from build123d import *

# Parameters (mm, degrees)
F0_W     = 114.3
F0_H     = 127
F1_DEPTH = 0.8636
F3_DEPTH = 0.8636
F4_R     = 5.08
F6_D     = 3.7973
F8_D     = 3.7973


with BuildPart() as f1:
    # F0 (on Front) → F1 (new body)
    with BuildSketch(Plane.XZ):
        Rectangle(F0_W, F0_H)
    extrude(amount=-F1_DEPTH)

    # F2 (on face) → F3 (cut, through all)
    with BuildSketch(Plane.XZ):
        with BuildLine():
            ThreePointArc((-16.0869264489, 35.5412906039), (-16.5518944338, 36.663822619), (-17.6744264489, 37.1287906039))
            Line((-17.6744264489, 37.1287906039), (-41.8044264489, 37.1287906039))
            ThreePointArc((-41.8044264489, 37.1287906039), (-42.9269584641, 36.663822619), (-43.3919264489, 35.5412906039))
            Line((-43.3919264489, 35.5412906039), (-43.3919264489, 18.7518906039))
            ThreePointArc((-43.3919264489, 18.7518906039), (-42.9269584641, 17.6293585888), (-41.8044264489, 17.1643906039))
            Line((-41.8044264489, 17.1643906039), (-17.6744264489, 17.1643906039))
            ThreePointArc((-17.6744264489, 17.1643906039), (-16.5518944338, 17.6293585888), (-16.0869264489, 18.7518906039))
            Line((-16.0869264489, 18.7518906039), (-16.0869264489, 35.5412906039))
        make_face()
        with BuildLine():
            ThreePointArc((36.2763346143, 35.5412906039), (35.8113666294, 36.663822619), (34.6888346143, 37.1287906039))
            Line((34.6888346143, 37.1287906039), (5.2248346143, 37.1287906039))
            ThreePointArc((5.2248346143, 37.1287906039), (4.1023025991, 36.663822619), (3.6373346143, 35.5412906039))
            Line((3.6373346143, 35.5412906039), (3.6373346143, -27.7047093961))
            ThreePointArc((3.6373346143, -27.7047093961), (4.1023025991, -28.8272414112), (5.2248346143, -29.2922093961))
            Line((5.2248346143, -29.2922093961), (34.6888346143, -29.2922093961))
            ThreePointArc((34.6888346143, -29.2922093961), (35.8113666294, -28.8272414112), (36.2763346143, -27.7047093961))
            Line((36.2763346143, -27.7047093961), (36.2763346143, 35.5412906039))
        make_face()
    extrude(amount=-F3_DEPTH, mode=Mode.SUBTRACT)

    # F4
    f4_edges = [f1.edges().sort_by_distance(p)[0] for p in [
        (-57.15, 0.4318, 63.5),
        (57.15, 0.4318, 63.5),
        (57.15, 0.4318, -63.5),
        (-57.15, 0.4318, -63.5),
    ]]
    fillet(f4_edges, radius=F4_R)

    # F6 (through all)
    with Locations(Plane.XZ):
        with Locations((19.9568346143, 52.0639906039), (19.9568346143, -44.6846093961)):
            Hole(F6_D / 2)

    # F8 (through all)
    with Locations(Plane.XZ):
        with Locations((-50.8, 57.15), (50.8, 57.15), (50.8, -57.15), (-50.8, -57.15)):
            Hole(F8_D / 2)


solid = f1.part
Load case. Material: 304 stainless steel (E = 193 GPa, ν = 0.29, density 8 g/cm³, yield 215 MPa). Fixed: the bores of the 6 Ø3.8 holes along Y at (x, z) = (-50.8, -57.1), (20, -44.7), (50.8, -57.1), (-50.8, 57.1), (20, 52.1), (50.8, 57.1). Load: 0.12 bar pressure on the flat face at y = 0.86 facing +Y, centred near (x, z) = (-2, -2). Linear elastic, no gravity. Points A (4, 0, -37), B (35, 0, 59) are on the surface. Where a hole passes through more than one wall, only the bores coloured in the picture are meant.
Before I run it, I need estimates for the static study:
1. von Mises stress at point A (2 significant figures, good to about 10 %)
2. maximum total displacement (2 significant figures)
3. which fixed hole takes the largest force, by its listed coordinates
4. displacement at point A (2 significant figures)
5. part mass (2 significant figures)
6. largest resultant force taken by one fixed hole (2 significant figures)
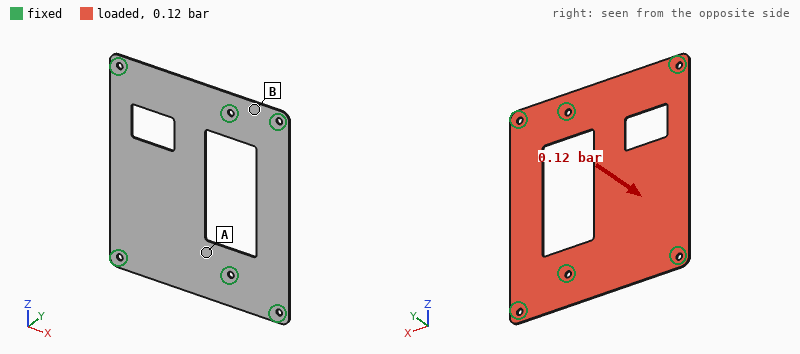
33 MPa
0.60 mm
(20, -44.7)
0.13 mm
81 g
38 N
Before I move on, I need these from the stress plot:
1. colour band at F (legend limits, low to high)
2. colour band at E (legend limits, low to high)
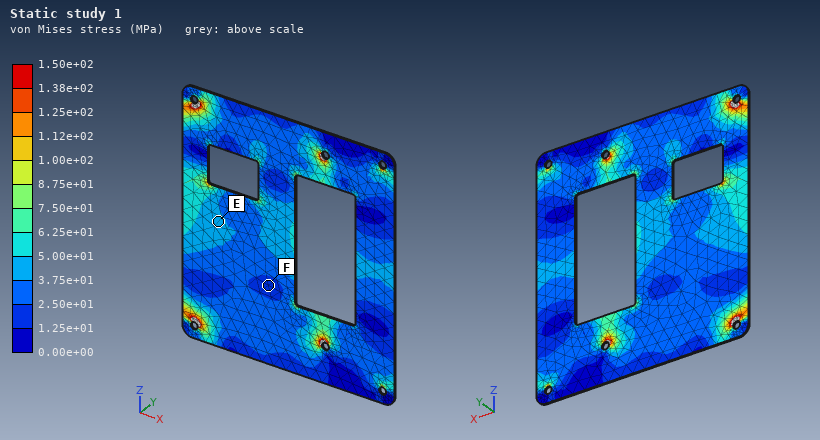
1.25e+01 to 2.50e+01 MPa
3.75e+01 to 5.00e+01 MPa
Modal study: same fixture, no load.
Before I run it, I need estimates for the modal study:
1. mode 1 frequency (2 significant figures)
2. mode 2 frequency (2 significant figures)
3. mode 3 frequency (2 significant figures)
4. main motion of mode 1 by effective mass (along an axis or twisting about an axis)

320 Hz
420 Hz
580 Hz
along Y
